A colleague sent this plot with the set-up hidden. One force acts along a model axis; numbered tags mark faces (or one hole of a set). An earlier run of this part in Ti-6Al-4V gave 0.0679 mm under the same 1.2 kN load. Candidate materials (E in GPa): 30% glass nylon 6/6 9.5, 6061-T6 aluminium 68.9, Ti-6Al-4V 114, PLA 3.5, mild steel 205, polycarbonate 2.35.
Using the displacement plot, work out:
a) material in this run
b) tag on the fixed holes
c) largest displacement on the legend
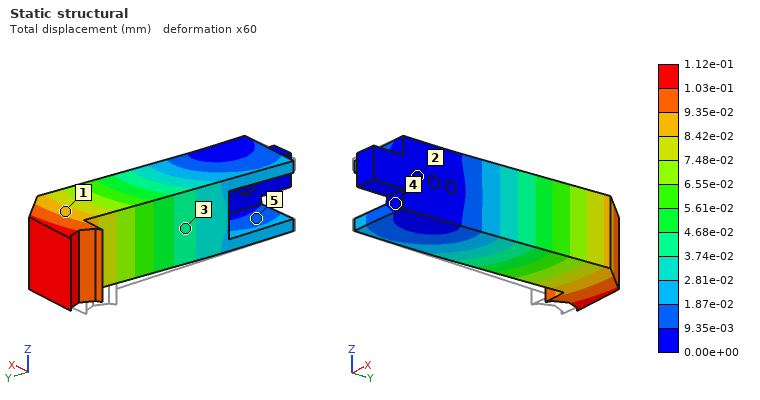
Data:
6061-T6 aluminium
2
1.12e-01 mm
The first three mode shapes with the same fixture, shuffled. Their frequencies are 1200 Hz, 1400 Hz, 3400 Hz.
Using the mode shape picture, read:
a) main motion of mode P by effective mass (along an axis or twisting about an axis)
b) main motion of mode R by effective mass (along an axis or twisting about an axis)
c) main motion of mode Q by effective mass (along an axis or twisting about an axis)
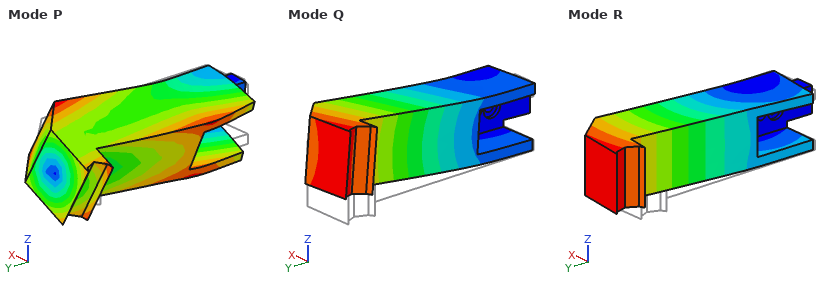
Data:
twisting about Y
along X
along Z
